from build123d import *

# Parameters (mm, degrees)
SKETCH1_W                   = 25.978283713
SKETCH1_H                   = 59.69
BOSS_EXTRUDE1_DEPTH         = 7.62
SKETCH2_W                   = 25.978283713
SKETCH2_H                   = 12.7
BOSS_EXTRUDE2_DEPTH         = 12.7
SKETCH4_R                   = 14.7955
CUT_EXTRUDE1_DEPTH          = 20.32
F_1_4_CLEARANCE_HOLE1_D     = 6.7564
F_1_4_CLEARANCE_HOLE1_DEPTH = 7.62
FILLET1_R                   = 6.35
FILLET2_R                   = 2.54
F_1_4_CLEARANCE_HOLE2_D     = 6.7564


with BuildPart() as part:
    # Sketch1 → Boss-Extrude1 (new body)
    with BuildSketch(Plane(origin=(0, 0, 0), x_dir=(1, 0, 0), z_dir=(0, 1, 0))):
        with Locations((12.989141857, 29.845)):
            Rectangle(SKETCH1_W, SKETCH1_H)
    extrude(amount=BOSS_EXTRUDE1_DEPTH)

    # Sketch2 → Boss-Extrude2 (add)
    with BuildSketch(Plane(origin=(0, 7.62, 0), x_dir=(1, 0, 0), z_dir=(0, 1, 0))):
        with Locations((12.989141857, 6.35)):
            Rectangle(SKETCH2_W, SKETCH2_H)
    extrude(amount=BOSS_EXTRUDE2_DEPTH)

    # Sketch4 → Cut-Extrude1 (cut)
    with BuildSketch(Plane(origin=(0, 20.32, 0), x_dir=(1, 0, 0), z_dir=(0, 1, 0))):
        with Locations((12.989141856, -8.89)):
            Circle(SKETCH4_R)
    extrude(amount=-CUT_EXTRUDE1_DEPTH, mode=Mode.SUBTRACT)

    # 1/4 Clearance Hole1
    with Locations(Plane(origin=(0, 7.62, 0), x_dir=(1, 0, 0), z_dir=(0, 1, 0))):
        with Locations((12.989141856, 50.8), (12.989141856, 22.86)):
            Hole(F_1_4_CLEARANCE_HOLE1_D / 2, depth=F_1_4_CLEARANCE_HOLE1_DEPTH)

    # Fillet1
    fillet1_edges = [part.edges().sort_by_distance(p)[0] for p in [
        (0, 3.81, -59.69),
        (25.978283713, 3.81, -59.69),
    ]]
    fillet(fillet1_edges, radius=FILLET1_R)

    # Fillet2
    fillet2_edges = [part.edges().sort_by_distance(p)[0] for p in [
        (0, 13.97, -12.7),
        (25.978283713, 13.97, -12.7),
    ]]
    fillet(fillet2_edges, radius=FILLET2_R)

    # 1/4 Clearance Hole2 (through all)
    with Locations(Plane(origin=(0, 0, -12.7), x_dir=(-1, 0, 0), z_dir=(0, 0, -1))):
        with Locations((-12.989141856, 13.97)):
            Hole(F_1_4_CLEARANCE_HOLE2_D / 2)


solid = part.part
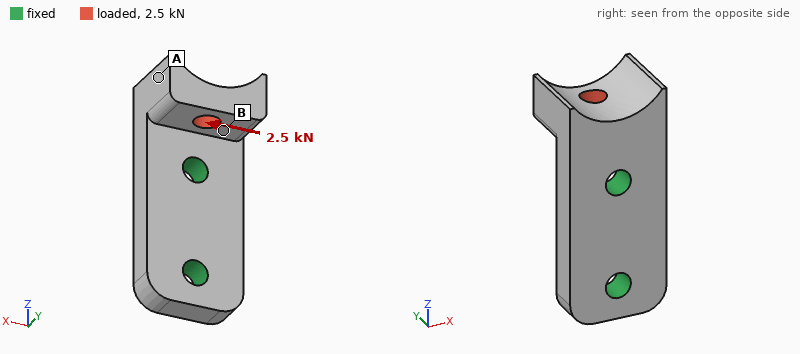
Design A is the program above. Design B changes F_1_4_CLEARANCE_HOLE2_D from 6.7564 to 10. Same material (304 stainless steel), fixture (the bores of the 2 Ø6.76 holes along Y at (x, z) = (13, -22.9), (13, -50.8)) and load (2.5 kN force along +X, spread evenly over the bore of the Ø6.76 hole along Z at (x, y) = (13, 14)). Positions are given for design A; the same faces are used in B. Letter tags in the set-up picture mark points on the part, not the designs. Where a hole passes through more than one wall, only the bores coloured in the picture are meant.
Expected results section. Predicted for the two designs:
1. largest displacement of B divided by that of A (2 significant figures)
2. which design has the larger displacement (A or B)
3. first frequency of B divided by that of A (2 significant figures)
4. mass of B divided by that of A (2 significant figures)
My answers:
1.1
B
1.0
0.98
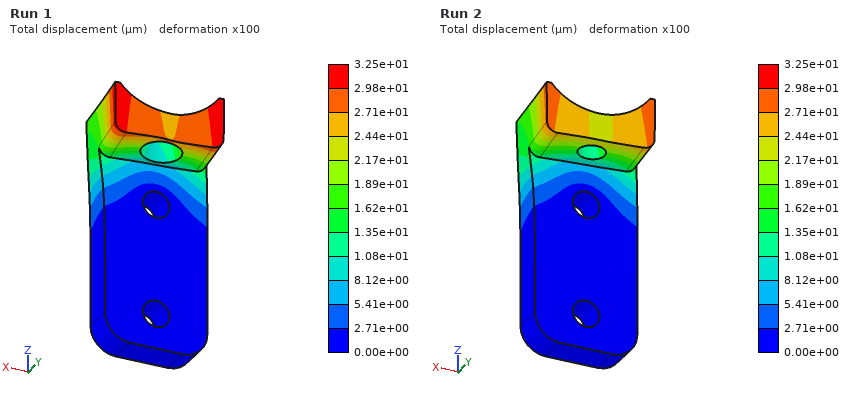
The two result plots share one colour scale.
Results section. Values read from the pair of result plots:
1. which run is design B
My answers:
Run 1
